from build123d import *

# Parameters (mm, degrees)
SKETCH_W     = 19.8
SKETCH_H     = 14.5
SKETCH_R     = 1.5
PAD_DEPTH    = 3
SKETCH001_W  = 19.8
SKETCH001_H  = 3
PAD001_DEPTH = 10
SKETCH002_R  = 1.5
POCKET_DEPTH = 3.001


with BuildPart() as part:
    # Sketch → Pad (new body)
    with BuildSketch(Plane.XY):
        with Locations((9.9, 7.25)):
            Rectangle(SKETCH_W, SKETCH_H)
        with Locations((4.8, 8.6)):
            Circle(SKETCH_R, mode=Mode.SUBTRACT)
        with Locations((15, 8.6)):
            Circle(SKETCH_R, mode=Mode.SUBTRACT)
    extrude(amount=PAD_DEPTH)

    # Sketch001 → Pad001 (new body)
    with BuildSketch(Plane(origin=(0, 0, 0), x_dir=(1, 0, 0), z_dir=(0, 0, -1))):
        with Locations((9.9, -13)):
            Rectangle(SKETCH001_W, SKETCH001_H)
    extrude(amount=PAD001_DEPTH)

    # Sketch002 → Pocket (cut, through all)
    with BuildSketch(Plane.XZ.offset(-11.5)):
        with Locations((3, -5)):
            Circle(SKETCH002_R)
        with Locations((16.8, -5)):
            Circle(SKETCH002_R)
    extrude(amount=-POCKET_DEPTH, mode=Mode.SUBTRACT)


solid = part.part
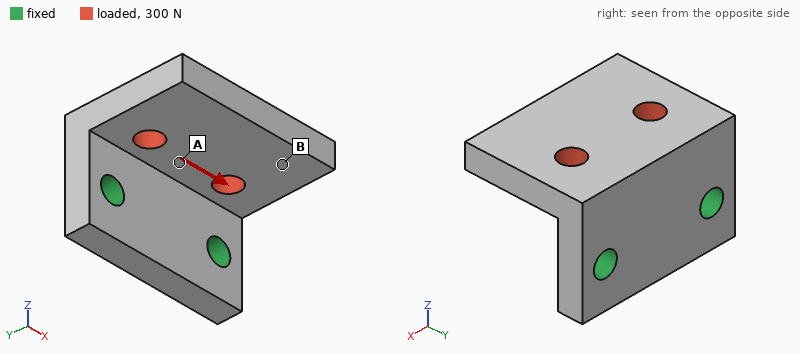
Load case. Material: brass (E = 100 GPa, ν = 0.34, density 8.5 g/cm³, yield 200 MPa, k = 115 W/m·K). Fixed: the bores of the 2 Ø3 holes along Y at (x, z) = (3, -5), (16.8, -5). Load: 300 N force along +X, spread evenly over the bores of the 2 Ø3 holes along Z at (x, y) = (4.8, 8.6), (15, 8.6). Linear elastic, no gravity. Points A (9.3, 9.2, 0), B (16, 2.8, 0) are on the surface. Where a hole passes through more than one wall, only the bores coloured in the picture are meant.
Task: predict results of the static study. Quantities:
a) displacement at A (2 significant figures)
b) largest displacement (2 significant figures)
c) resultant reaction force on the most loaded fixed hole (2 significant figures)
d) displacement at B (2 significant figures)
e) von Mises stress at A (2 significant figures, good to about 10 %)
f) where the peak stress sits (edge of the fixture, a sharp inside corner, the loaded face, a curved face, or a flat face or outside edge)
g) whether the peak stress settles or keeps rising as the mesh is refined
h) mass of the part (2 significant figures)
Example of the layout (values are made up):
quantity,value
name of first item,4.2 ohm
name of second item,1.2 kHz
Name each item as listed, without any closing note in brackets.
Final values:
quantity,value
displacement at A,2.5 µm
largest displacement,6.7 µm
resultant reaction force on the most loaded fixed hole,210 N
displacement at B,5.3 µm
von Mises stress at A,14 MPa
where the peak stress sits,edge of the fixture
whether the peak stress settles or keeps rising as the mesh is refined,keeps rising
mass of the part,12 g
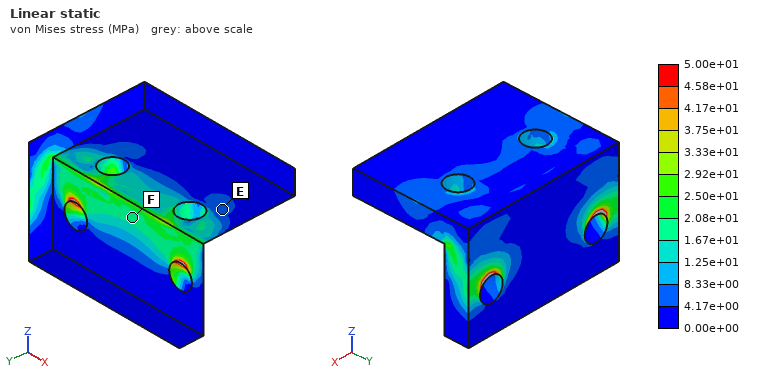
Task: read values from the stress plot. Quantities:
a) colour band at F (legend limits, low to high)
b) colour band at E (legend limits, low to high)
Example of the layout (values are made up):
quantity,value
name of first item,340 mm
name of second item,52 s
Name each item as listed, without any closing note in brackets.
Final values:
quantity,value
colour band at F,1.67e+01 to 2.08e+01 MPa
colour band at E,4.17e+00 to 8.33e+00 MPa
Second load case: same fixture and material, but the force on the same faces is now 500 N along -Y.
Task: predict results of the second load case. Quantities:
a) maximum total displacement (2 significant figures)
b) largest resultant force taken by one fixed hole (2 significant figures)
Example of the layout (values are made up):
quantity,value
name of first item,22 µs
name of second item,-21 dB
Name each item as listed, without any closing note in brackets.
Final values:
quantity,value
maximum total displacement,31 µm
largest resultant force taken by one fixed hole,250 N
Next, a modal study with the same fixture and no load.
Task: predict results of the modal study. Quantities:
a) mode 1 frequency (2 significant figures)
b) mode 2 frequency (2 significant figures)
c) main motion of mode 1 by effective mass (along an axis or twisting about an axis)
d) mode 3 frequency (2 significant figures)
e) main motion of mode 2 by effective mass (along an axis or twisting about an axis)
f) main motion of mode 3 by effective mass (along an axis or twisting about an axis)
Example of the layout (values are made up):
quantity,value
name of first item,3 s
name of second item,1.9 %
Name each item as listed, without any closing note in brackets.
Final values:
quantity,value
mode 1 frequency,5700 Hz
mode 2 frequency,11 kHz
main motion of mode 1 by effective mass,along Z
mode 3 frequency,16 kHz
main motion of mode 2 by effective mass,along X
main motion of mode 3 by effective mass,along X
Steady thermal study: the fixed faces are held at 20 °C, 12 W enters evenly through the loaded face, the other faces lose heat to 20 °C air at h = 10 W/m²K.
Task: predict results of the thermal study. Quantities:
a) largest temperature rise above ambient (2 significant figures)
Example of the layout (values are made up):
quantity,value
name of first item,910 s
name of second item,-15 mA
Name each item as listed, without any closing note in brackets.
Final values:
quantity,value
largest temperature rise above ambient,20 K
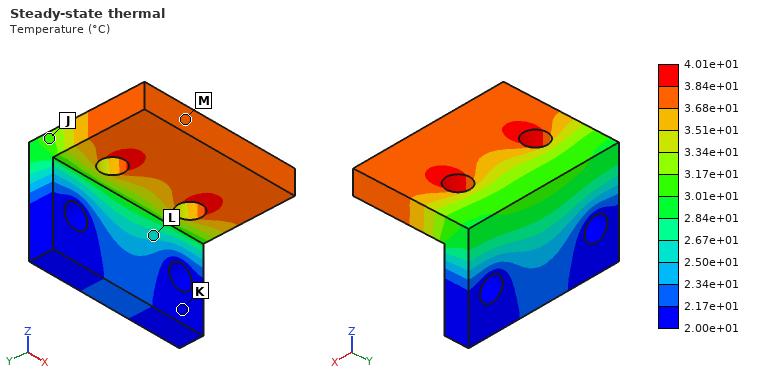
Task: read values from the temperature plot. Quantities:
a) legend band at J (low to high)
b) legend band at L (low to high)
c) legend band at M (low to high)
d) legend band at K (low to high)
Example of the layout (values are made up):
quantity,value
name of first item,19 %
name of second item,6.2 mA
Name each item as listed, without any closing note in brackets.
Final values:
quantity,value
legend band at J,3.01e+01 to 3.17e+01 °C
legend band at L,2.50e+01 to 2.67e+01 °C
legend band at M,3.68e+01 to 3.84e+01 °C
legend band at K,2.00e+01 to 2.17e+01 °C
